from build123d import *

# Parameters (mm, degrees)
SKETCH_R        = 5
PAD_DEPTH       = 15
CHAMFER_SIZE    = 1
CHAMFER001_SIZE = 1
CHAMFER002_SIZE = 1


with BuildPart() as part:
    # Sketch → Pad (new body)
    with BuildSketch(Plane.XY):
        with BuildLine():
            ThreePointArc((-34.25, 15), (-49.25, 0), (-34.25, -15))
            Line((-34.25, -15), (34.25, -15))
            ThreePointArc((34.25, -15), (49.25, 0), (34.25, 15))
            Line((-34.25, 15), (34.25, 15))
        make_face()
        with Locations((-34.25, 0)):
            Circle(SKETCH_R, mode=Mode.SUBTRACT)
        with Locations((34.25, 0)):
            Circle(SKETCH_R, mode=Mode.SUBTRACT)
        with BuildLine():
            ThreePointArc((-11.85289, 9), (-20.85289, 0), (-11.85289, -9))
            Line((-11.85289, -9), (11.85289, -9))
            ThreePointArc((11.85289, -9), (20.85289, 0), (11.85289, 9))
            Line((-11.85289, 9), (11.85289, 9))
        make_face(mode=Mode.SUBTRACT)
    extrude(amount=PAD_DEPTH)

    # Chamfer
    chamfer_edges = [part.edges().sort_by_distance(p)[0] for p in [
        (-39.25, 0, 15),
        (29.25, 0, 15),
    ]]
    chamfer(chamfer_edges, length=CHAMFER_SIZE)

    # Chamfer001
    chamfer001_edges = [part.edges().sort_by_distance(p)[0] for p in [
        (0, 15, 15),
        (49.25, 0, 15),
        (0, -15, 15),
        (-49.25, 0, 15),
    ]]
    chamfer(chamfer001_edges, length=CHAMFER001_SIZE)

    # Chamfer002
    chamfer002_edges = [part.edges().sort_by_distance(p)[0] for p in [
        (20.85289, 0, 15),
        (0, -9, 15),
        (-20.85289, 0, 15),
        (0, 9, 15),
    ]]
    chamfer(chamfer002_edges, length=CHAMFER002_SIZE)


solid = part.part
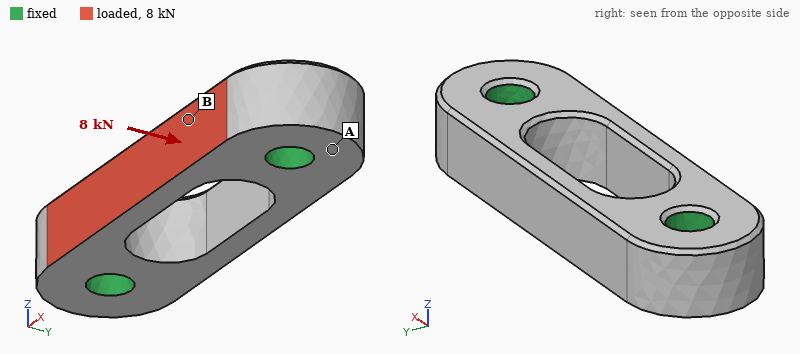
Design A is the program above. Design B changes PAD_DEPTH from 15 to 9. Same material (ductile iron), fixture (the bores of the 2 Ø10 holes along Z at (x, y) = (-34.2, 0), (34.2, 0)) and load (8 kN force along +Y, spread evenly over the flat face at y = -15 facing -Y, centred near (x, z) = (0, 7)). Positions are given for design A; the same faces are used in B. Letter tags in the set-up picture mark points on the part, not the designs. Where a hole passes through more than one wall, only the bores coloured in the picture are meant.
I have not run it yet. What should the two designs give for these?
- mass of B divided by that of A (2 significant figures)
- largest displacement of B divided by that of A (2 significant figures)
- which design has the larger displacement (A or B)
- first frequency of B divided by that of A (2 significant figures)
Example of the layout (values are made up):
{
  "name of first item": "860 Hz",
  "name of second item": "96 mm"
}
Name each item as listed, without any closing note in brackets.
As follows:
{
  "mass of B divided by that of A": "0.60",
  "largest displacement of B divided by that of A": "1.7",
  "which design has the larger displacement": "B",
  "first frequency of B divided by that of A": "0.74"
}
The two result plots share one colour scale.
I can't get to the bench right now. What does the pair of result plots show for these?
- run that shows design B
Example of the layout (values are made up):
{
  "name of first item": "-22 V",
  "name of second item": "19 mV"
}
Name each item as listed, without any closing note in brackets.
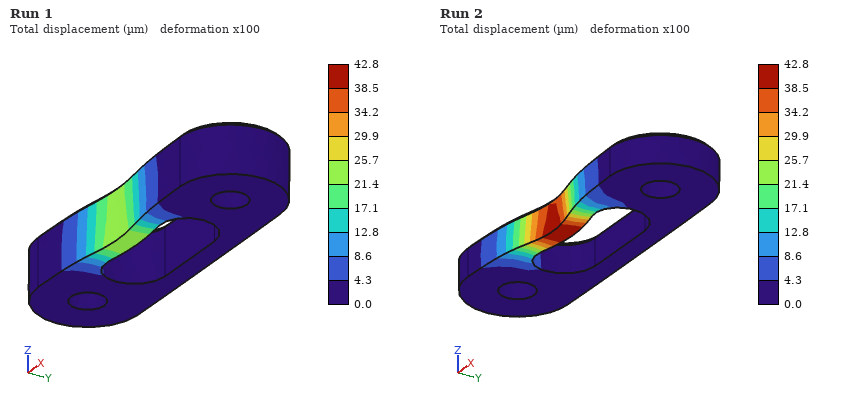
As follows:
{
  "run that shows design B": "Run 2"
}
